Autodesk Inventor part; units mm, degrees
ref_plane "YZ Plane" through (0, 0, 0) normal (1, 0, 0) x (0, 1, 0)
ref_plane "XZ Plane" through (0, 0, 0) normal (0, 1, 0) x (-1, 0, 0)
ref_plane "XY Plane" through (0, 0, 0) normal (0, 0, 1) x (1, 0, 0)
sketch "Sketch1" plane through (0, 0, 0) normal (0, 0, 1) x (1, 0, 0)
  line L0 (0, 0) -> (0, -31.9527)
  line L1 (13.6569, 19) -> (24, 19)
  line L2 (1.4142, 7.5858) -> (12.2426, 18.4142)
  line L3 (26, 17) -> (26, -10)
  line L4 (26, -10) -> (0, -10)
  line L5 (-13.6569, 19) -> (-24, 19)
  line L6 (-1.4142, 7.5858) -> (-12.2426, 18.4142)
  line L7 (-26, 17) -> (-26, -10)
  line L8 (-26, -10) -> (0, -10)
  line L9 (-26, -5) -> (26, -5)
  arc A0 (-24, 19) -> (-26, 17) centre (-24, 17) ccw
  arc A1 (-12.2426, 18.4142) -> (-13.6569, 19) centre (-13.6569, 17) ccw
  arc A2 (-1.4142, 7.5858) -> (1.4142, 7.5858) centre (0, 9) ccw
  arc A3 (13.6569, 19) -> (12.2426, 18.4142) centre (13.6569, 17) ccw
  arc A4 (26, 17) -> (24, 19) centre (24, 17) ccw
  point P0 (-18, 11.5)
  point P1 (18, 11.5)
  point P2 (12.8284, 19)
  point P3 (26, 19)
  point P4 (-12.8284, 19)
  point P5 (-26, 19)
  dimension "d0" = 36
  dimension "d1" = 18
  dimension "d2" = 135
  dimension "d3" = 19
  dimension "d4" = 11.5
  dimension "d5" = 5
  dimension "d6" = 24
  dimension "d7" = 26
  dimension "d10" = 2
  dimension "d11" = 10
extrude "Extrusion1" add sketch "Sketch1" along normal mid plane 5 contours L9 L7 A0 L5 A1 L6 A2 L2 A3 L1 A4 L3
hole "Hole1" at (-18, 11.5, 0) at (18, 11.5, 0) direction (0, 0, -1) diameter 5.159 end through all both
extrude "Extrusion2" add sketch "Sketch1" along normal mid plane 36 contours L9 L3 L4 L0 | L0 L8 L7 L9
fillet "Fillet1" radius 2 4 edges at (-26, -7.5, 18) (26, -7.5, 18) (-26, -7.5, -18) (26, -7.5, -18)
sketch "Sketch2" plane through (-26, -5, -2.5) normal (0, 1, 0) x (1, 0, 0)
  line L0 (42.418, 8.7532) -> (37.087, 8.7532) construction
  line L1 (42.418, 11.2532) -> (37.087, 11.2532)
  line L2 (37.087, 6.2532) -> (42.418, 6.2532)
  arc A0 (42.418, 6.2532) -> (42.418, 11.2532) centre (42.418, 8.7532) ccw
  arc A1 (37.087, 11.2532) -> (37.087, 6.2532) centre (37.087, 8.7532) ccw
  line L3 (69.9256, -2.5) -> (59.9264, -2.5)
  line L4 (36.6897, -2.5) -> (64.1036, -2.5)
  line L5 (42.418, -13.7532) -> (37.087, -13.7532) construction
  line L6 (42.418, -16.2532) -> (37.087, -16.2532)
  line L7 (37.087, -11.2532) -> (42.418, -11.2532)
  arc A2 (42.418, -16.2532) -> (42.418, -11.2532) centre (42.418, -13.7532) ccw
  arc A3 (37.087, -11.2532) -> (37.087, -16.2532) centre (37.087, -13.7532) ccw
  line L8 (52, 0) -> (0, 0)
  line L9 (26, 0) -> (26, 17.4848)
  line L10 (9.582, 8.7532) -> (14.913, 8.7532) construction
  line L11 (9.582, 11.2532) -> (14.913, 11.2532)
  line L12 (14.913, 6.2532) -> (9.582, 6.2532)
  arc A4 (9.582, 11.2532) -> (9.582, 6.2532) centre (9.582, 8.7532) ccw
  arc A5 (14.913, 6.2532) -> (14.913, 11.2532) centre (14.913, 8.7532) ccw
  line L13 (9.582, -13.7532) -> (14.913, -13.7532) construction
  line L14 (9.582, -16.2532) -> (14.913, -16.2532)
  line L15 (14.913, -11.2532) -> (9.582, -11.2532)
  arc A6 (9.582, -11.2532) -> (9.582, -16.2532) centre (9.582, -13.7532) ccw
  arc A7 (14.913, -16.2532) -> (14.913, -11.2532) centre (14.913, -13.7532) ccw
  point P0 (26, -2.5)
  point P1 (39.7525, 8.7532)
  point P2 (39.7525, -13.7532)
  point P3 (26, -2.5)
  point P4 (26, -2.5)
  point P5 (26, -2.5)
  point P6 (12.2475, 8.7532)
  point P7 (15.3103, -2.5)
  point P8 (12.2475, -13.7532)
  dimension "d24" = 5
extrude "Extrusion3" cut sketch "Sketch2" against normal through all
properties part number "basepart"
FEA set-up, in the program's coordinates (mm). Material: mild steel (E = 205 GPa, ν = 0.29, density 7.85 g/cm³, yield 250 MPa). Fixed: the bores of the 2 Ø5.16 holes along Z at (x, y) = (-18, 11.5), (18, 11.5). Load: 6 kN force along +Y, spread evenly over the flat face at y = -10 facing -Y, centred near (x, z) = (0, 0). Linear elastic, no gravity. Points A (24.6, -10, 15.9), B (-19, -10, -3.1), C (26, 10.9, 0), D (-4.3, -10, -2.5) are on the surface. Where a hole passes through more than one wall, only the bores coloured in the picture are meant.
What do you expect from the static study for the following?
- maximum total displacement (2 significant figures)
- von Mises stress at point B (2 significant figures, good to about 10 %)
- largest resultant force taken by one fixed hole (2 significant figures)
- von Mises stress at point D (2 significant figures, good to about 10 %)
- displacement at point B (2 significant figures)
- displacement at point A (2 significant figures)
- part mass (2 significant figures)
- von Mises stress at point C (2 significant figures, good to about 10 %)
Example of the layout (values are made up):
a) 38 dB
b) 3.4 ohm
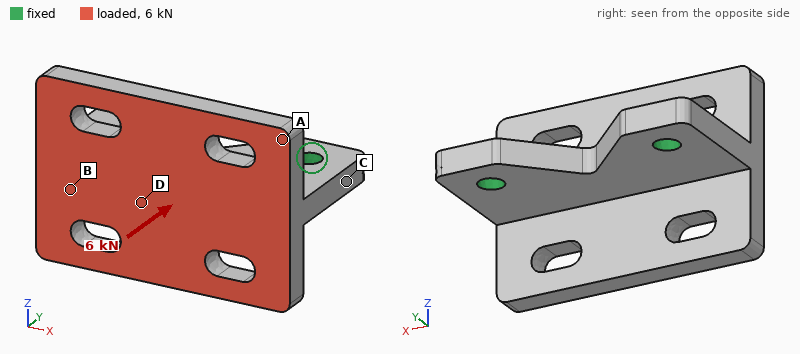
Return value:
a) 23 µm
b) 72 MPa
c) 3.1 kN
d) 81 MPa
e) 3.4 µm
f) 18 µm
g) 110 g
h) 18 MPa
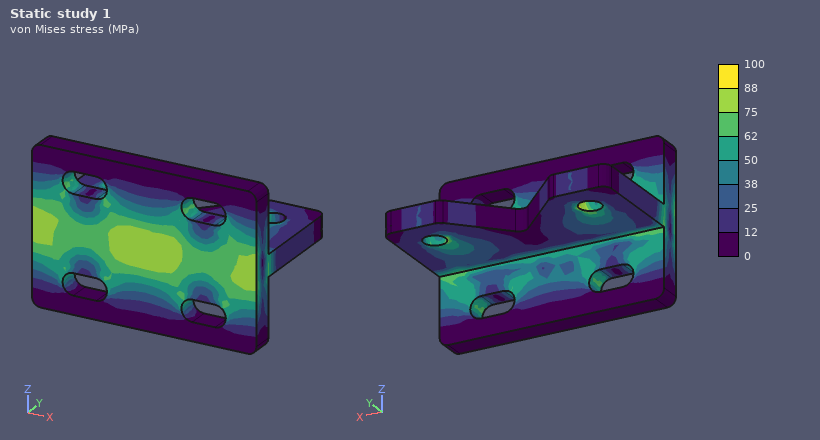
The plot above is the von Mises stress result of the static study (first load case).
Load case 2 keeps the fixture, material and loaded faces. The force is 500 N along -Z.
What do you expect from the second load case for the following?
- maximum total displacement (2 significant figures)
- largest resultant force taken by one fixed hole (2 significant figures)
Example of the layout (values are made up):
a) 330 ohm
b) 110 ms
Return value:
a) 27 µm
b) 250 N
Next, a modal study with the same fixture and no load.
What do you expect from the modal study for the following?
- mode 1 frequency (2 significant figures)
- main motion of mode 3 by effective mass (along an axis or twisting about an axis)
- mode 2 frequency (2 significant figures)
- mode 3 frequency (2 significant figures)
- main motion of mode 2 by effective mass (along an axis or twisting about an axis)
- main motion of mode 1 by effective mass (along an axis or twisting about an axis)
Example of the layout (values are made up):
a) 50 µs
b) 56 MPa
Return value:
a) 3000 Hz
b) along Z
c) 5700 Hz
d) 9600 Hz
e) twisting about Y
f) along Z
